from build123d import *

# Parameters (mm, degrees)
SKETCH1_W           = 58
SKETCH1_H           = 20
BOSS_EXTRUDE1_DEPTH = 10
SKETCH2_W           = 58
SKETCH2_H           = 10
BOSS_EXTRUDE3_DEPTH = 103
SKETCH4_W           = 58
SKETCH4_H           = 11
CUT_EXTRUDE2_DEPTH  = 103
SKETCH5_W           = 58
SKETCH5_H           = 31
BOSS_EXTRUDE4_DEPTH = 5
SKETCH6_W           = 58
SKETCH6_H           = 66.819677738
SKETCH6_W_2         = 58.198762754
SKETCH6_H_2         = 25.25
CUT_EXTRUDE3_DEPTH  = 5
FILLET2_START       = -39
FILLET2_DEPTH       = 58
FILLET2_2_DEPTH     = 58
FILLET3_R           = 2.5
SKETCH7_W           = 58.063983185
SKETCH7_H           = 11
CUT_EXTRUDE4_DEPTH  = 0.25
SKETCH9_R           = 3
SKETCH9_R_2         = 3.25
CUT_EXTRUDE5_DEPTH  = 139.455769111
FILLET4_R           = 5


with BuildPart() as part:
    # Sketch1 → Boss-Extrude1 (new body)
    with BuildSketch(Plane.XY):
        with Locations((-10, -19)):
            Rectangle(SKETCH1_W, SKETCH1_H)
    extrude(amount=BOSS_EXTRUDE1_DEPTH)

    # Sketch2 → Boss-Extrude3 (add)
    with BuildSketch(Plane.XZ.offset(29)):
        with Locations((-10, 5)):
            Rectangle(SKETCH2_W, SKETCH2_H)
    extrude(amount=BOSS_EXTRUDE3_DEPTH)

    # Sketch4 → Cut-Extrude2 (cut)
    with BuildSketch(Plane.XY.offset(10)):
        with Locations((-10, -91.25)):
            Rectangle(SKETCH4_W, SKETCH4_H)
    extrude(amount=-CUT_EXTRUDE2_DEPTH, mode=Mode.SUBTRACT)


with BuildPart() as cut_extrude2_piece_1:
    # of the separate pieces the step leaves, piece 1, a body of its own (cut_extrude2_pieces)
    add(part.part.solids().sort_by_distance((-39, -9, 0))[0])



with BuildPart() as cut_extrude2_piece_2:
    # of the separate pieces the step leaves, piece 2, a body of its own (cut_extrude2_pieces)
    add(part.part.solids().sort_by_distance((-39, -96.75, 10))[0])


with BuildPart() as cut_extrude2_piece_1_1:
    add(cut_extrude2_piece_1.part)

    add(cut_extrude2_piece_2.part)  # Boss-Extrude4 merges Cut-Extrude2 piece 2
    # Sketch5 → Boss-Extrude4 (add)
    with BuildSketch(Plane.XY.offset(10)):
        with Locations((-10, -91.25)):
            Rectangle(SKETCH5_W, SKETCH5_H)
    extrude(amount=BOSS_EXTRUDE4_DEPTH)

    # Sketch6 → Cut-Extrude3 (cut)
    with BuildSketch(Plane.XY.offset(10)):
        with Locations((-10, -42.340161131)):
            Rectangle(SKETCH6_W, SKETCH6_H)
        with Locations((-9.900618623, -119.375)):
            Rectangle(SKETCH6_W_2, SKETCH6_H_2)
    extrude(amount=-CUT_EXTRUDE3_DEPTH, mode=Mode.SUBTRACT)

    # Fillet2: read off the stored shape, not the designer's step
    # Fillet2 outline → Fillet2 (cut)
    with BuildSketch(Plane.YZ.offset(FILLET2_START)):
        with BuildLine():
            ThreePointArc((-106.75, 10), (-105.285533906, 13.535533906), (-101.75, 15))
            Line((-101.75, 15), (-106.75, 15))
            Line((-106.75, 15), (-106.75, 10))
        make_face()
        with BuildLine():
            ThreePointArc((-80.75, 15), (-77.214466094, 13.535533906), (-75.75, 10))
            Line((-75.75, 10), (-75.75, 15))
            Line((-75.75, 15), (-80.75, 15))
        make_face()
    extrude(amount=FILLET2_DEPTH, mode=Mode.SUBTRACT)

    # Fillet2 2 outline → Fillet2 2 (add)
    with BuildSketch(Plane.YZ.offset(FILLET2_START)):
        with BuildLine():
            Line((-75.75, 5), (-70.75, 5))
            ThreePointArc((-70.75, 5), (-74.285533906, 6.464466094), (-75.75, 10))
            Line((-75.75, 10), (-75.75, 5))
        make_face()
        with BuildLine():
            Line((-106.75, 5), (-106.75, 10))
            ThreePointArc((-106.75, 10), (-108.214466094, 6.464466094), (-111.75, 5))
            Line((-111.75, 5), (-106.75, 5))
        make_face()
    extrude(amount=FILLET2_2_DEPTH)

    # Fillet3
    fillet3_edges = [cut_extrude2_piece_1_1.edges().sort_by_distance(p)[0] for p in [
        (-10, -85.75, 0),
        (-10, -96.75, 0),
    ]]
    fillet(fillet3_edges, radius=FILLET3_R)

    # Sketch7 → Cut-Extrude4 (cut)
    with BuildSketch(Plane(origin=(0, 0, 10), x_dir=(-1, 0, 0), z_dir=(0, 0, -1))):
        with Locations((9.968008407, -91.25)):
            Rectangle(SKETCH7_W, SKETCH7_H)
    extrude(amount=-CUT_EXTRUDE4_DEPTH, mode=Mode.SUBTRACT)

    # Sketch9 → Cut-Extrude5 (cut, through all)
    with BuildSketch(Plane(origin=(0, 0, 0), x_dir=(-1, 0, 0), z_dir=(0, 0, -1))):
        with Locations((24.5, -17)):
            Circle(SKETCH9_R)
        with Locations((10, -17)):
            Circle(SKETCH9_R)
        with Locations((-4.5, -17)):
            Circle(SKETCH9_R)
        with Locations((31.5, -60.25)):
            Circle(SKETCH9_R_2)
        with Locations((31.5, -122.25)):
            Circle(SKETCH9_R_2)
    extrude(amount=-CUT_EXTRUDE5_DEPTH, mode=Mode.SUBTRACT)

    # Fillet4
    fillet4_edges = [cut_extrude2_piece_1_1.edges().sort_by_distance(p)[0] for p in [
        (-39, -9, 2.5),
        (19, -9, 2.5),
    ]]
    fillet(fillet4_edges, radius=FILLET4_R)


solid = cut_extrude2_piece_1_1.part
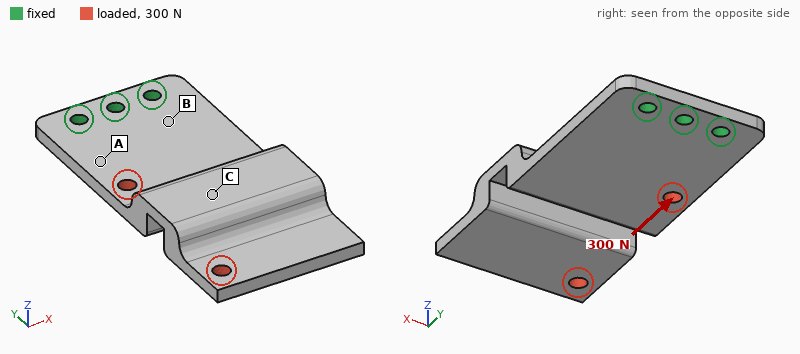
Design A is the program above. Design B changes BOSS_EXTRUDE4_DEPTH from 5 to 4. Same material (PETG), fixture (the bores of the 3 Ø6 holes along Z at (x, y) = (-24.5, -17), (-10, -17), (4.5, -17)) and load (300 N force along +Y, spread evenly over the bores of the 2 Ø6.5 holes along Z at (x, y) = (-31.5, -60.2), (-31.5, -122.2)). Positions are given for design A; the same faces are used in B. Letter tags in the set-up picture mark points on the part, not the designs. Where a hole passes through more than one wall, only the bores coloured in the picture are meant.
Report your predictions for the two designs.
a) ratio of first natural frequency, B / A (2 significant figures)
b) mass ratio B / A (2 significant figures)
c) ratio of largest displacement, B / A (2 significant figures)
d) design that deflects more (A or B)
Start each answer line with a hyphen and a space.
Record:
- 1.0
- 0.97
- 1.6
- B
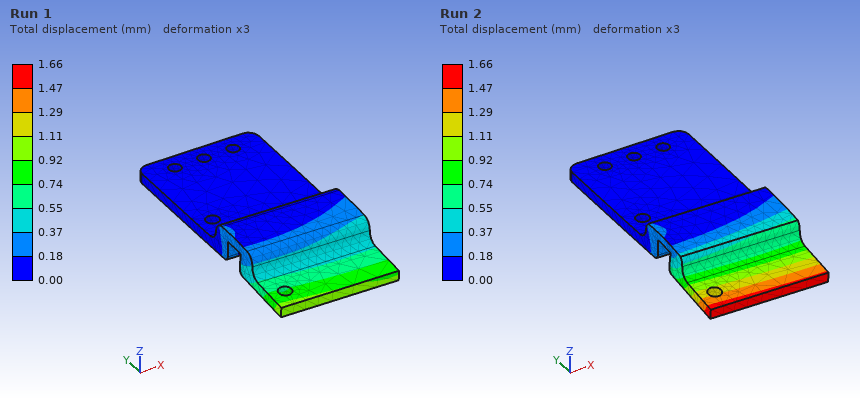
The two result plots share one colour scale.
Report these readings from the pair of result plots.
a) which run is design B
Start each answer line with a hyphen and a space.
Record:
- Run 2
